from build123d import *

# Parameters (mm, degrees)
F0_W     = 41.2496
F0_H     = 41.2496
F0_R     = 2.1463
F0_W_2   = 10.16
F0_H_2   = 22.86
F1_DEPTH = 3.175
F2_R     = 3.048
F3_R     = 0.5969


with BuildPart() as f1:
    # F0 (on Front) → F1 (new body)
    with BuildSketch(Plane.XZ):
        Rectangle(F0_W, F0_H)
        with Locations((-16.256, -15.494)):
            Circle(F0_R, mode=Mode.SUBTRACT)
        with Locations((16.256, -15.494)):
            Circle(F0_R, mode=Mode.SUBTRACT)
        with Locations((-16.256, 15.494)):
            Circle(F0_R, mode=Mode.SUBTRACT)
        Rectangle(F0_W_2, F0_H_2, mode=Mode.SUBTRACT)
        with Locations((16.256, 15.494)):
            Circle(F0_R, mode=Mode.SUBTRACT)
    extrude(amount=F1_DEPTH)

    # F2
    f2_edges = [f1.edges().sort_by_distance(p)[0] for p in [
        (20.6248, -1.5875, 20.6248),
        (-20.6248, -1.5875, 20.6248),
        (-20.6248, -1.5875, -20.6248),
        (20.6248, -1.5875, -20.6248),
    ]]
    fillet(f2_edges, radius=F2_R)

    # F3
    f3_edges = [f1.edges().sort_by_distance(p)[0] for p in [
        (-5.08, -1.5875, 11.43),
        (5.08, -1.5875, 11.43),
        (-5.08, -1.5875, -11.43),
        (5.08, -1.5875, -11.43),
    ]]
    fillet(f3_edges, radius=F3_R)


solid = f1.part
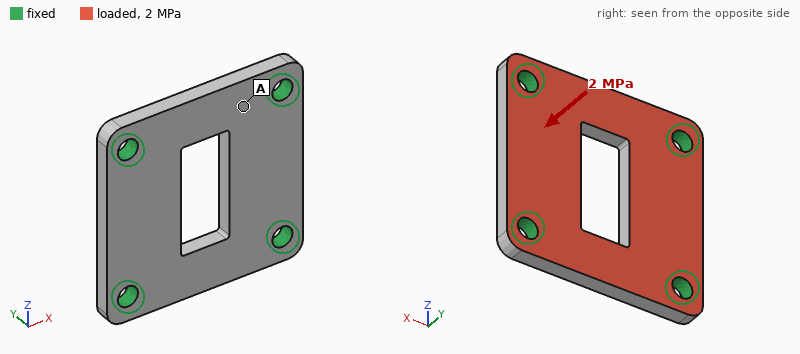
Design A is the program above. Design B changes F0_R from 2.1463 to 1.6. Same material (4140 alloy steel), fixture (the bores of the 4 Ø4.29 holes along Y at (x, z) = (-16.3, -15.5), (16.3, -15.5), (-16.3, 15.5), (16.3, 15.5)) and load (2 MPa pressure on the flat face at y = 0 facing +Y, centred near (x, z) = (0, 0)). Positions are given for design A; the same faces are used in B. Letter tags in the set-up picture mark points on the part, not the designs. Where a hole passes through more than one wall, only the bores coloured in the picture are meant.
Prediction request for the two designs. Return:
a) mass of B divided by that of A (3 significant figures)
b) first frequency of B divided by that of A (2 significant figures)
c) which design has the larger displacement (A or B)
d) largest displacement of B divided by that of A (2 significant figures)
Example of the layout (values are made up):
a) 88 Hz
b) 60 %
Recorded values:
a) 1.02
b) 0.91
c) B
d) 1.2
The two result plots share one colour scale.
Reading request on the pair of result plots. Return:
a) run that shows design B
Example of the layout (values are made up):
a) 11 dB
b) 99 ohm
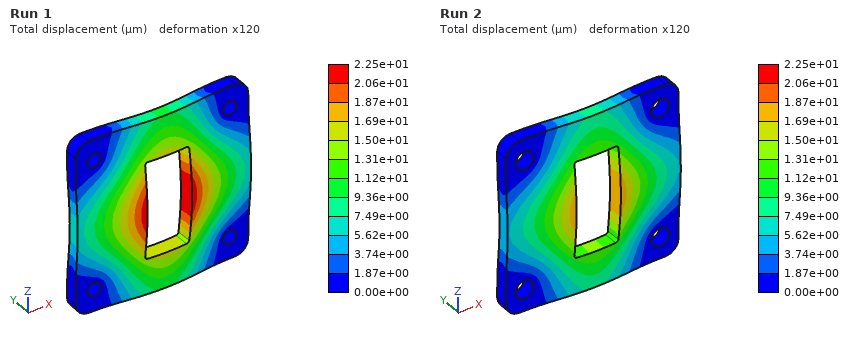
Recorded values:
a) Run 1
